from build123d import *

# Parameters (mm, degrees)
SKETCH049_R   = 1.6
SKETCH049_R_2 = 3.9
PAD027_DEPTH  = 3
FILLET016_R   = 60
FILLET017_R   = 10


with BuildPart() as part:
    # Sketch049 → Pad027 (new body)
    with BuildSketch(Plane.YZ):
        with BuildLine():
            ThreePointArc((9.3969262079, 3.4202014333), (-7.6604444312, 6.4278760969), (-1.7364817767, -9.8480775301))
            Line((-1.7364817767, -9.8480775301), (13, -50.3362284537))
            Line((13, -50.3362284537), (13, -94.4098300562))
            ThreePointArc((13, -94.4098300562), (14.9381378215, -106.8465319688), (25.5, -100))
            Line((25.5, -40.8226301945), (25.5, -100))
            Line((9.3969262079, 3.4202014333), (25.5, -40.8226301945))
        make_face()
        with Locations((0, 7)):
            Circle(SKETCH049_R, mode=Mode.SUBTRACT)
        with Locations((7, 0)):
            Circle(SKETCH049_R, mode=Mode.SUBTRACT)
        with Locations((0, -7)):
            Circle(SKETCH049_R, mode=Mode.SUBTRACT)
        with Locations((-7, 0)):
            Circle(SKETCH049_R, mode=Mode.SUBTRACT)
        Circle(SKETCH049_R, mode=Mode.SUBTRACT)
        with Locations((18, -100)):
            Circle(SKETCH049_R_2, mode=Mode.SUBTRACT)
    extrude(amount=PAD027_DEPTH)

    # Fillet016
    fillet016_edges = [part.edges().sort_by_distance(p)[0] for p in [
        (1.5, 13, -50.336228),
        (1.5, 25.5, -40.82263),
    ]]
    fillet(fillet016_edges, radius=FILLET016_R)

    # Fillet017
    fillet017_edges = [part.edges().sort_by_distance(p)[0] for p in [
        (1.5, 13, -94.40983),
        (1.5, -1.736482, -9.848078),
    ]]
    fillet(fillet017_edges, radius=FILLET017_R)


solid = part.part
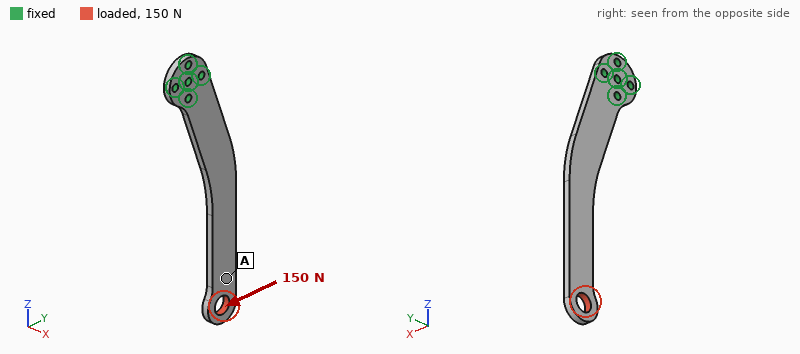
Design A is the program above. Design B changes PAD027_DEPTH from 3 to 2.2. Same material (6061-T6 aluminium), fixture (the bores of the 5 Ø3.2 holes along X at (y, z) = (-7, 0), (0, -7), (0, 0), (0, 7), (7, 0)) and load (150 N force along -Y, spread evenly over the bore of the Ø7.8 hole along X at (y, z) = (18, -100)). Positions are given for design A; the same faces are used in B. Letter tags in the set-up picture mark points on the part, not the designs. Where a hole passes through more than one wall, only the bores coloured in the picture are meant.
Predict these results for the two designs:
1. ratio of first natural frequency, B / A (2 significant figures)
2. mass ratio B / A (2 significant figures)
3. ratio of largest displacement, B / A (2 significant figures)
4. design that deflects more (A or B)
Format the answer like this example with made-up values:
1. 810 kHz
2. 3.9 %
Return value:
1. 0.74
2. 0.73
3. 1.4
4. B
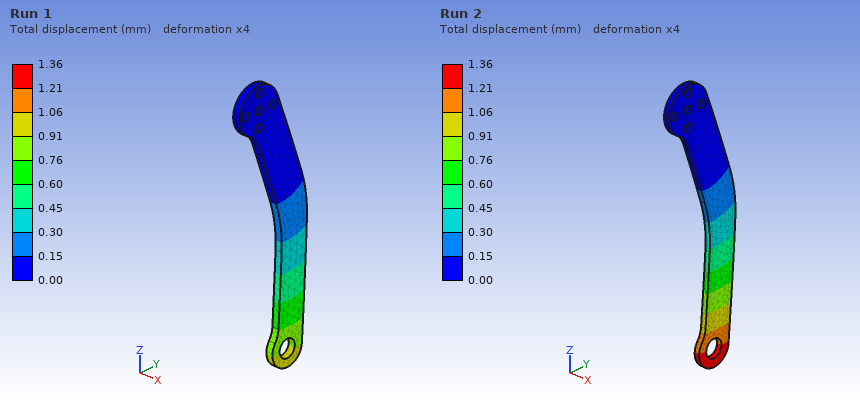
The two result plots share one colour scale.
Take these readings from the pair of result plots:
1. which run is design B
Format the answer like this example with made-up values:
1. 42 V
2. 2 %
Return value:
1. Run 2
